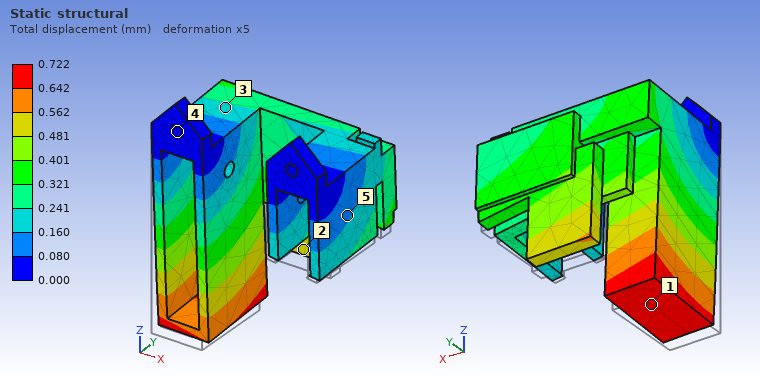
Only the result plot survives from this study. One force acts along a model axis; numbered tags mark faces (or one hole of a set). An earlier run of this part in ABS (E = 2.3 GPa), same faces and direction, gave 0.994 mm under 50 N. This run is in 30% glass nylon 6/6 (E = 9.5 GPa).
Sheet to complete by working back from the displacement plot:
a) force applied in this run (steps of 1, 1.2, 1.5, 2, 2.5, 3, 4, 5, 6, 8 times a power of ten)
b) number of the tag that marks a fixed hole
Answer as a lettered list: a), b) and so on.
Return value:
a) 150 N
b) 4
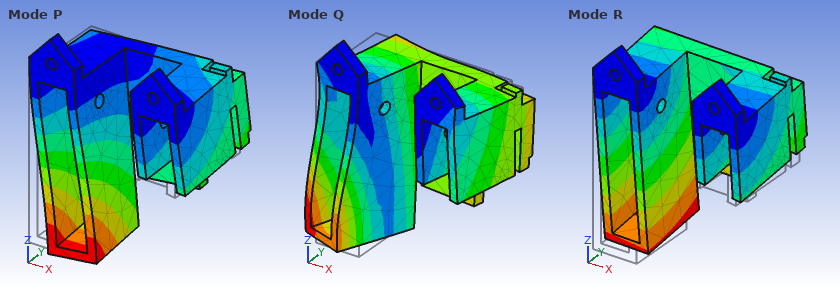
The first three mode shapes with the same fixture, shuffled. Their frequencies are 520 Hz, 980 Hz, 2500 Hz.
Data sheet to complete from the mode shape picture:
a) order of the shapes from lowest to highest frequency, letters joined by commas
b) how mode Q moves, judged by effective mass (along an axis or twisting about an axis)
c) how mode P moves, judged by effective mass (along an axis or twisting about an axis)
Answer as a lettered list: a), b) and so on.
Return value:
a) R, P, Q
b) along X
c) along X
